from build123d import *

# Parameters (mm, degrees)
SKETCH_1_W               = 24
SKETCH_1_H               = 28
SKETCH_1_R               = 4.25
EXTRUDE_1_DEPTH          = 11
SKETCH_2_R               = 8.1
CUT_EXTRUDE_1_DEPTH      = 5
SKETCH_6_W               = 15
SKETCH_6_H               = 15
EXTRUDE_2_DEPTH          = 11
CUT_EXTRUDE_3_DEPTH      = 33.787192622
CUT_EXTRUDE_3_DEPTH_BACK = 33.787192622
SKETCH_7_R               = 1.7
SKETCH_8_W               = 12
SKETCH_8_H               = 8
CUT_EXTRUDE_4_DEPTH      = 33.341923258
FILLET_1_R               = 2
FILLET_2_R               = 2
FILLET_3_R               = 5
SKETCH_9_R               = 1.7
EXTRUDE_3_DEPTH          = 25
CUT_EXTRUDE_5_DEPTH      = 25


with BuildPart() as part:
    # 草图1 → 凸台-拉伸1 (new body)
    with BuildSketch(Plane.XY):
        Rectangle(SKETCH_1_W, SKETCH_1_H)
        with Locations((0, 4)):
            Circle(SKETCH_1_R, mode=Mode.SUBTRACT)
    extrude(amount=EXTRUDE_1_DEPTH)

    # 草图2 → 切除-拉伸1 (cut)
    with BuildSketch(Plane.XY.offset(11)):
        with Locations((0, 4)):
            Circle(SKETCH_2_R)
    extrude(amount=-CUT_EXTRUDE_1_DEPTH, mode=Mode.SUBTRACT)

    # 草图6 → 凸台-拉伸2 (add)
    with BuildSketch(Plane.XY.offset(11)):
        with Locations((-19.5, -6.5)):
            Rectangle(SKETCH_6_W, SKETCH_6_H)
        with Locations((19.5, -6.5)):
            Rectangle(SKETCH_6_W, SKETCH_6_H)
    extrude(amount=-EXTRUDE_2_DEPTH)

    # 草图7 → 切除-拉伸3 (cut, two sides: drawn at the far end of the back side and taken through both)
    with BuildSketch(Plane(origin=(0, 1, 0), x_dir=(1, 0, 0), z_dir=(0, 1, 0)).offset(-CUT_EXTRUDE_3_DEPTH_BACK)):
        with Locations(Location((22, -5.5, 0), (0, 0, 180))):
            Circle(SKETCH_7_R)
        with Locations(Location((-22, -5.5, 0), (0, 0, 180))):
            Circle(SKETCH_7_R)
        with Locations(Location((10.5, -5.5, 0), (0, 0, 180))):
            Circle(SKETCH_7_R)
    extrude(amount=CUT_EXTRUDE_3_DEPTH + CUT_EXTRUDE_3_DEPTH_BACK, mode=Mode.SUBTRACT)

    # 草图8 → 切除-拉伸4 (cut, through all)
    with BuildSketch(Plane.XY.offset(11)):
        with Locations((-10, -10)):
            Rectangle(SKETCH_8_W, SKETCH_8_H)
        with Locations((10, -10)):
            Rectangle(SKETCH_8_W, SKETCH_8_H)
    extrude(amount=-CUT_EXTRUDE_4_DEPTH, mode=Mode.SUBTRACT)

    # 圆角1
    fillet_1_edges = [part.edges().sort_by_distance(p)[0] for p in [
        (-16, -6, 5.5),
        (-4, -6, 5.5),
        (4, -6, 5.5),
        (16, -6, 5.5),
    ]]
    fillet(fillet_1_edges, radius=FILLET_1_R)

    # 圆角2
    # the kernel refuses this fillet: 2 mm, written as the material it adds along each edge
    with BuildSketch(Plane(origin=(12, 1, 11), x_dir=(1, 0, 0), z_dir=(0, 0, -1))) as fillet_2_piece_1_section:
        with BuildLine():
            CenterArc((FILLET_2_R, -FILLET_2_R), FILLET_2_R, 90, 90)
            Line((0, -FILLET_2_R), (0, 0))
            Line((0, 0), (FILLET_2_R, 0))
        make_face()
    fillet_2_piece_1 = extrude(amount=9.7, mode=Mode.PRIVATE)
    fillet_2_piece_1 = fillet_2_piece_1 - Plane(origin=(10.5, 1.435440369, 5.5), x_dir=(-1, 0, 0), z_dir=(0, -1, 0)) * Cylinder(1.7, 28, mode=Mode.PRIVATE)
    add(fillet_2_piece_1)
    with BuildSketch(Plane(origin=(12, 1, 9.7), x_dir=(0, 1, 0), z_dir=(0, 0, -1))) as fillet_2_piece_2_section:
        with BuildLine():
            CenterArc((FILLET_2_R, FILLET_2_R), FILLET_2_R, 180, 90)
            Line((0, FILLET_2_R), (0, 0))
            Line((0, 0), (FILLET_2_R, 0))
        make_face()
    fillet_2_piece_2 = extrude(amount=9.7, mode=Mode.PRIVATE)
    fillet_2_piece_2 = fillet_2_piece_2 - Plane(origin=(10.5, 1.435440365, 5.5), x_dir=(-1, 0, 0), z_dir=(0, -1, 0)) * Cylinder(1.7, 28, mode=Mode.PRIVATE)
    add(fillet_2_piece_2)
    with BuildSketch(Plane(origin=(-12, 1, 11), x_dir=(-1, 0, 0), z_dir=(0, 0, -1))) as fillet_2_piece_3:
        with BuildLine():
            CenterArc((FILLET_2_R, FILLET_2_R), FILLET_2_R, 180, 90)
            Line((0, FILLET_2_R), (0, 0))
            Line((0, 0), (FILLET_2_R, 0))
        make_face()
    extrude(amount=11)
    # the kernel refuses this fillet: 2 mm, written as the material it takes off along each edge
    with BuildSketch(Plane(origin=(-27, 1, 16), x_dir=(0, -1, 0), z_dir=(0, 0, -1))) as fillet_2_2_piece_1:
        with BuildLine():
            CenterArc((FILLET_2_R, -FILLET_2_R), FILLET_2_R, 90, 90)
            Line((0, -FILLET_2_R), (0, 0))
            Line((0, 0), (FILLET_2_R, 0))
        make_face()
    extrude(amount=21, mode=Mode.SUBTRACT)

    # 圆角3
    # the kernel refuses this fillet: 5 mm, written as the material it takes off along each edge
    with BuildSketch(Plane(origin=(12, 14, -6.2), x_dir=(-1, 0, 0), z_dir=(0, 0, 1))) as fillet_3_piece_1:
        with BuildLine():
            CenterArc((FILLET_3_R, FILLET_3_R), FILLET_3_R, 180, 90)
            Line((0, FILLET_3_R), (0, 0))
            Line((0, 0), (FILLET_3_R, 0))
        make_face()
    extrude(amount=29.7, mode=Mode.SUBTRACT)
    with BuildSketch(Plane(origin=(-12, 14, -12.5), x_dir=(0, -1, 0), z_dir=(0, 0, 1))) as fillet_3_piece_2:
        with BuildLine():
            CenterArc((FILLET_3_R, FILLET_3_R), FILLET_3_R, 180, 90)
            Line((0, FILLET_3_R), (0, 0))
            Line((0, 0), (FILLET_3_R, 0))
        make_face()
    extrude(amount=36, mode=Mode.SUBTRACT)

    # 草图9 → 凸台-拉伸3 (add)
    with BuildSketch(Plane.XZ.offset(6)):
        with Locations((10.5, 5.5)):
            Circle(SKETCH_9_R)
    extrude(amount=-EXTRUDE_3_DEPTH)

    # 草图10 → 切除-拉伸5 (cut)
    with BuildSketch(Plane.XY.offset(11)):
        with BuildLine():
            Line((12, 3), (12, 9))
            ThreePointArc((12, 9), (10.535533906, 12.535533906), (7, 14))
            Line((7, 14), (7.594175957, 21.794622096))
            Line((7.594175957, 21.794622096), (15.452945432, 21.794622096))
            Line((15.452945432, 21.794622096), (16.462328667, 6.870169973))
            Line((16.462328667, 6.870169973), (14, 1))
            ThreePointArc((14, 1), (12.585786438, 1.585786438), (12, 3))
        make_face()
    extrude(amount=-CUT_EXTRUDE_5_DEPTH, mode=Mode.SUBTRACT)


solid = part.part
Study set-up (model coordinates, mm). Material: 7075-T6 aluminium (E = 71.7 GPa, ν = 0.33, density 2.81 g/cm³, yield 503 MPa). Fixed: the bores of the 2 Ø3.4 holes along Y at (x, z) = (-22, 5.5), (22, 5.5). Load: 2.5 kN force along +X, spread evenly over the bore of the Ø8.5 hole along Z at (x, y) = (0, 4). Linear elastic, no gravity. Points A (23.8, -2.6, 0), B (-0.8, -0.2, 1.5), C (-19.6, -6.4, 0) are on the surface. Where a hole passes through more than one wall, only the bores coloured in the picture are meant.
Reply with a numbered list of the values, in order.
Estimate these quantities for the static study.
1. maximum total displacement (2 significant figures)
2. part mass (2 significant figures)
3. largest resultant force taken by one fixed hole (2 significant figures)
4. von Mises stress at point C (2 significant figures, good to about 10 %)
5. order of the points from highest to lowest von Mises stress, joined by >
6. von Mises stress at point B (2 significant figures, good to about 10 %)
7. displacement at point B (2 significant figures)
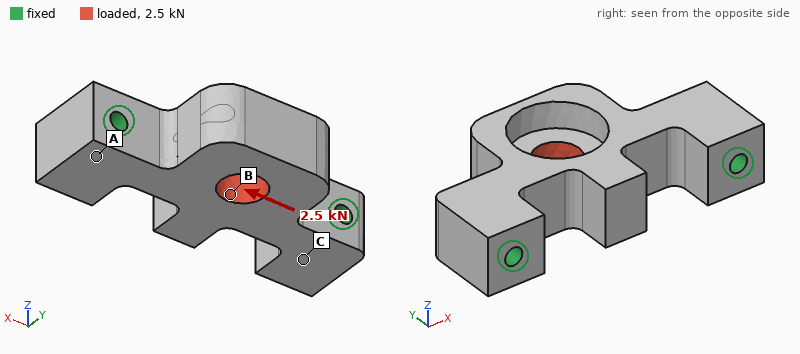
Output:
1. 11 µm
2. 24 g
3. 1.4 kN
4. 8.9 MPa
5. B > C > A
6. 29 MPa
7. 4.5 µm
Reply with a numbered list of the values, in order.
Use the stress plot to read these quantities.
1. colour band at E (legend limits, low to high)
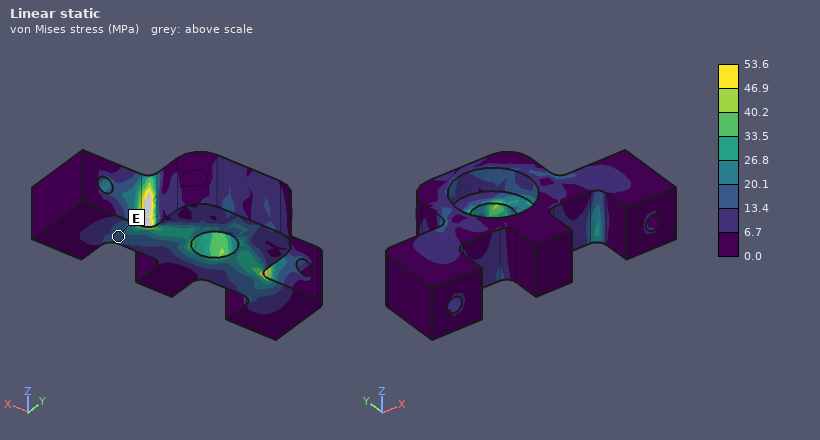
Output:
1. 13.4 to 20.1 MPa
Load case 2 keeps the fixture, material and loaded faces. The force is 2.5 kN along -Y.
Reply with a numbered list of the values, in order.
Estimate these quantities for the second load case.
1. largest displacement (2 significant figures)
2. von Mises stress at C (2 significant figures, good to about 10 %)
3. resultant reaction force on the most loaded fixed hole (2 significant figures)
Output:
1. 31 µm
2. 24 MPa
3. 1.3 kN
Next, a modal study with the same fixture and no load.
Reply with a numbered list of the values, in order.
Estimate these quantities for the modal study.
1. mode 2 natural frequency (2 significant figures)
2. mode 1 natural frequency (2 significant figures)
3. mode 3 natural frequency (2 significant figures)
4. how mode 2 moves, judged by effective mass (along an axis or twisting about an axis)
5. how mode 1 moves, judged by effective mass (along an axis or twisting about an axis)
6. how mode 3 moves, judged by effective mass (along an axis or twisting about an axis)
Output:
1. 14 kHz
2. 10000 Hz
3. 19 kHz
4. along Z
5. along Z
6. along Y
